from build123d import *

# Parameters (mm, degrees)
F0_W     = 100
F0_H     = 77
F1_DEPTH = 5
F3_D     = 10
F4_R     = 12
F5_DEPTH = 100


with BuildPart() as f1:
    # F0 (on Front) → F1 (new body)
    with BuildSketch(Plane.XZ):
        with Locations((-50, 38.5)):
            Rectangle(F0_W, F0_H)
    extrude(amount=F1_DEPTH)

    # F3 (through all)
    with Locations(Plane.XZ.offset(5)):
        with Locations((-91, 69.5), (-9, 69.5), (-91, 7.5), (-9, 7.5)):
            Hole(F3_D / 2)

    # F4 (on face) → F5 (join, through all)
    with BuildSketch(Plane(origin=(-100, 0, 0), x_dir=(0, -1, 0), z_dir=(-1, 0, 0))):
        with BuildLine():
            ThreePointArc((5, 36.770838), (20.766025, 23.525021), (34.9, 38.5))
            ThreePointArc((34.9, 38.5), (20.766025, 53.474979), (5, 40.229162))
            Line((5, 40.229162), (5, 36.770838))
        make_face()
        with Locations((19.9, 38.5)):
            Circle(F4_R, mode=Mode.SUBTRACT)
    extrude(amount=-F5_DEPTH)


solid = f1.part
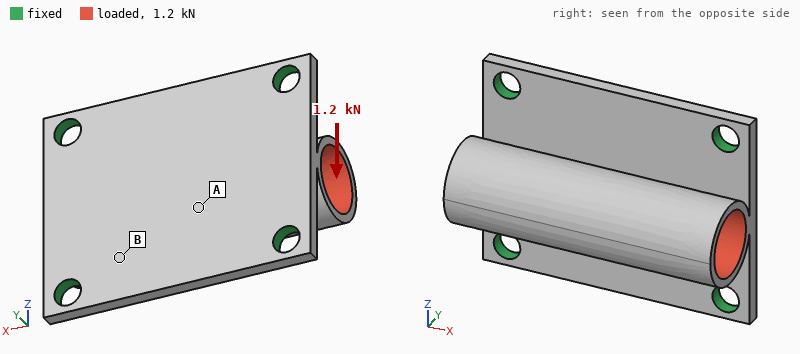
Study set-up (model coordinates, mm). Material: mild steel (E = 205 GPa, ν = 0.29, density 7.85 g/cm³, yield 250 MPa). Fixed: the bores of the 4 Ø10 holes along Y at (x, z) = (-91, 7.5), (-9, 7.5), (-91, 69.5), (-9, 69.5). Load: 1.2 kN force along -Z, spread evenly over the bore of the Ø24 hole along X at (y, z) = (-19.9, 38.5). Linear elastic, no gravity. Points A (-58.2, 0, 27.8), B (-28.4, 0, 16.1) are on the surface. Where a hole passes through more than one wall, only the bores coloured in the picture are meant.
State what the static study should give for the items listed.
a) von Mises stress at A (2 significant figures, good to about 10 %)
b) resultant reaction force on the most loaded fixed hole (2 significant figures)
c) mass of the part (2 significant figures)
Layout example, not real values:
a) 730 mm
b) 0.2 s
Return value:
a) 12 MPa
b) 390 N
c) 490 g
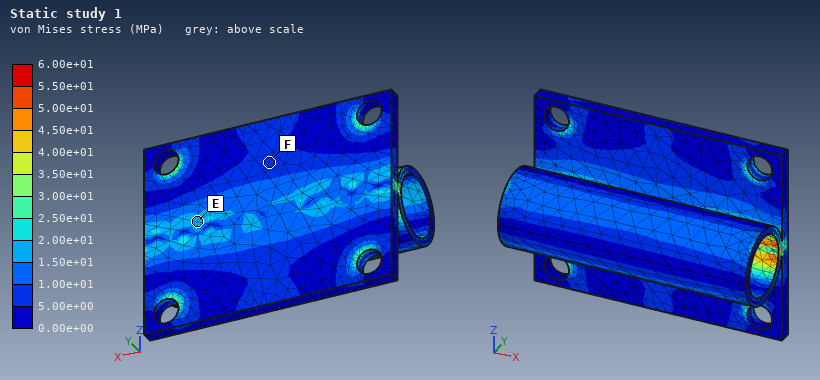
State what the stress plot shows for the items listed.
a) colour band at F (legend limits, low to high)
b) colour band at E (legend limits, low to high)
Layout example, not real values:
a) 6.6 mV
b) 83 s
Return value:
a) 5.00e+00 to 1.00e+01 MPa
b) 1.50e+01 to 2.00e+01 MPa
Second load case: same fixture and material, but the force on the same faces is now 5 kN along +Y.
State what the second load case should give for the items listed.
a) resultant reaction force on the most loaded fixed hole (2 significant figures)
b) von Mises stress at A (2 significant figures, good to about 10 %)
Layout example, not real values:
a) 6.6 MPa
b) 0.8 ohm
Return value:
a) 1.3 kN
b) 32 MPa
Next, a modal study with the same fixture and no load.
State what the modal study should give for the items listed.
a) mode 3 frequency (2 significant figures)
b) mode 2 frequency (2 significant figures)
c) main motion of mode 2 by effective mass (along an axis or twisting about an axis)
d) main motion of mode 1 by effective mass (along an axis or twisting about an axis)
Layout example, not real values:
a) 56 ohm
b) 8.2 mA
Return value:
a) 3500 Hz
b) 3000 Hz
c) along Y
d) along Z
